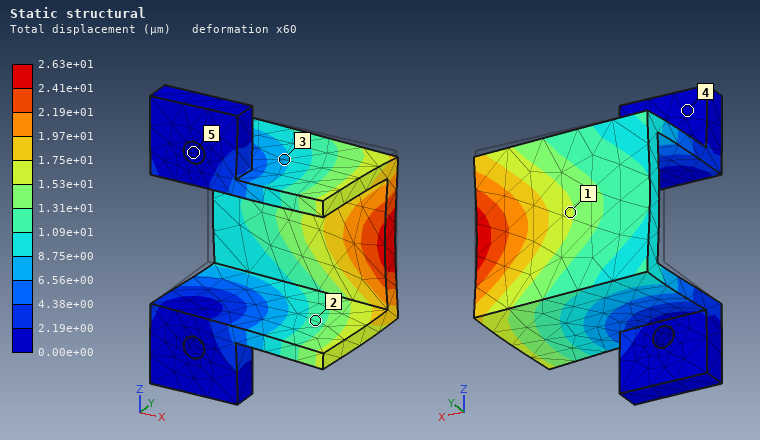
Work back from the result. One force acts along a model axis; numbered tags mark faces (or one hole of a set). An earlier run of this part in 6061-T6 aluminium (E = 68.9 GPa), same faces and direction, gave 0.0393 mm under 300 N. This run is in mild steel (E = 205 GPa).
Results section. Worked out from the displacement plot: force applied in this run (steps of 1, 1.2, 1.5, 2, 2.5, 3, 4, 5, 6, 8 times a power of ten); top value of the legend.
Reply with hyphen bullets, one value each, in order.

- 600 N
- 2.63e+01 µm
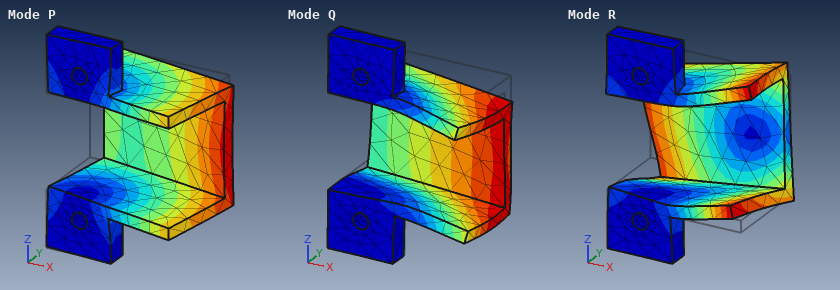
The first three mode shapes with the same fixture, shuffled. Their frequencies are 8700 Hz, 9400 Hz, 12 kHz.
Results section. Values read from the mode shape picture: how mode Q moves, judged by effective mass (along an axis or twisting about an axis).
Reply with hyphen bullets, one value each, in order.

- along Z
